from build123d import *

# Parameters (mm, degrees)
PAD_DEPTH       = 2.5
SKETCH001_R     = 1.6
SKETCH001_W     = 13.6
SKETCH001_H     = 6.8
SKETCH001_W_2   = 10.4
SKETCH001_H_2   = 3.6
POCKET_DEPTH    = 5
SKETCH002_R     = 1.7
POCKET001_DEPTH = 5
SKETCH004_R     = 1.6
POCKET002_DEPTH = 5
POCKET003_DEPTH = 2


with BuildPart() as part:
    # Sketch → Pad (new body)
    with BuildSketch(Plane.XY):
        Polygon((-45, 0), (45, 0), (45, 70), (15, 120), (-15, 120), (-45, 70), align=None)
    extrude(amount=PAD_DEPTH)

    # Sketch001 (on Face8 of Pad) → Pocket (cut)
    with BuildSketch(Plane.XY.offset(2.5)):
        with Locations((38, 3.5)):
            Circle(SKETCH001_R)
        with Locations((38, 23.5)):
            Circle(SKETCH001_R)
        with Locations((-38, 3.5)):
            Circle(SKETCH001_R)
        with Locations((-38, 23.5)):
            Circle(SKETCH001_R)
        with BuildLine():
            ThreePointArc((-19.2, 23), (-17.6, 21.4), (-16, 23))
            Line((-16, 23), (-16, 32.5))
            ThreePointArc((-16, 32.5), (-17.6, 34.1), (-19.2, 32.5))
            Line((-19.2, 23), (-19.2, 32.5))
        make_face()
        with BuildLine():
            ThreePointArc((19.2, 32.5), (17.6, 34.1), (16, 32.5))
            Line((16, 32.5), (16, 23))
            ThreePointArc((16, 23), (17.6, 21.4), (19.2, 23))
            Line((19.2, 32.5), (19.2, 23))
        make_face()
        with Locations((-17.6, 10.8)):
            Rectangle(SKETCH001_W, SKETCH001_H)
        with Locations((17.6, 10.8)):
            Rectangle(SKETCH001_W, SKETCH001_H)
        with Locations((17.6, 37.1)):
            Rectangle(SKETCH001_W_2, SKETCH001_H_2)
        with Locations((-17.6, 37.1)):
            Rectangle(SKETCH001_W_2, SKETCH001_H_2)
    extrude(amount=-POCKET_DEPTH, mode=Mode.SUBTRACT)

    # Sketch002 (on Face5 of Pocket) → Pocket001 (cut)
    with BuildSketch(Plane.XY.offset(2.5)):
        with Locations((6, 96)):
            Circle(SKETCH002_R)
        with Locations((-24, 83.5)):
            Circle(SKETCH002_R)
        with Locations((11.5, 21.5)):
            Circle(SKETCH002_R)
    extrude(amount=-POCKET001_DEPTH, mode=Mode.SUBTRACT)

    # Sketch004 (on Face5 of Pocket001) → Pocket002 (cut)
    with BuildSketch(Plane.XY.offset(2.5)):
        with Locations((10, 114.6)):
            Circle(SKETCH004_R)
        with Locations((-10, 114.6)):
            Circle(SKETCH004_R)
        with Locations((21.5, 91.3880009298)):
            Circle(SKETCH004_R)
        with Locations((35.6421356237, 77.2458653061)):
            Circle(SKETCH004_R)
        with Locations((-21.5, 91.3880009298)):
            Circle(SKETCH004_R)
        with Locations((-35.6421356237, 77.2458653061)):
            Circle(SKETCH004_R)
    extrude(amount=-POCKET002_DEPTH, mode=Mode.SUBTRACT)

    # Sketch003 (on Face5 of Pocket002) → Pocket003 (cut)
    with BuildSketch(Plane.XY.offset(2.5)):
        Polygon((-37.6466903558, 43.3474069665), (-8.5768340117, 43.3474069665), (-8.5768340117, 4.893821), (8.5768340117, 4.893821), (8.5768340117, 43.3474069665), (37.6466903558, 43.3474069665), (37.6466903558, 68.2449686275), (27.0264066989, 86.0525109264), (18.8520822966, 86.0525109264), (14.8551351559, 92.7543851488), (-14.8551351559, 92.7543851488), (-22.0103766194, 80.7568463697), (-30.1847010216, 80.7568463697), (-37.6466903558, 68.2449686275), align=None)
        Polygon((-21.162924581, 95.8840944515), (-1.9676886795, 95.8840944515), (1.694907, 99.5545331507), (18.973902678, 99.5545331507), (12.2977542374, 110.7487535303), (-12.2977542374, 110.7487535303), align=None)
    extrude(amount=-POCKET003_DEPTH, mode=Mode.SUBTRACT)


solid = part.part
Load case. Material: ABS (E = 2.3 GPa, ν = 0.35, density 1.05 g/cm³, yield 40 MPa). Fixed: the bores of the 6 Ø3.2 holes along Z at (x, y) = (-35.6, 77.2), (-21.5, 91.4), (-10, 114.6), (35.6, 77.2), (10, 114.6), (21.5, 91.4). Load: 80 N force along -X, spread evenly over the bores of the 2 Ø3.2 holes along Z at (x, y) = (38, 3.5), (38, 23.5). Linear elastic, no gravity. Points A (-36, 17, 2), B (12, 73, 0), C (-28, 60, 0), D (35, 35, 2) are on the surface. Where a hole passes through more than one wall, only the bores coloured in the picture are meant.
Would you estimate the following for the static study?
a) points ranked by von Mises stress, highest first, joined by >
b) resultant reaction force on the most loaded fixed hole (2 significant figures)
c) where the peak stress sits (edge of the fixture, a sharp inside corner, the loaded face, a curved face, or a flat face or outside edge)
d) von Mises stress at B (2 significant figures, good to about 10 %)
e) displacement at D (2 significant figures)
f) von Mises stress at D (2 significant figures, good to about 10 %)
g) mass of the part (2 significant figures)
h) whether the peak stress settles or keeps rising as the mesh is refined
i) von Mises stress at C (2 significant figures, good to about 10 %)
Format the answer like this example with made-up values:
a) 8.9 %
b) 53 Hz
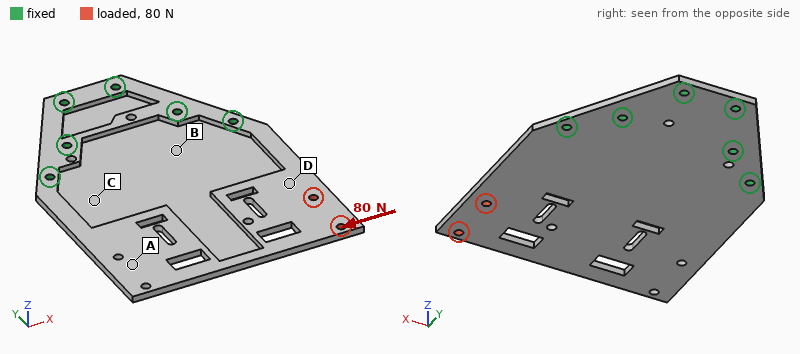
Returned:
a) C > B > D > A
b) 72 N
c) edge of the fixture
d) 3.0 MPa
e) 0.52 mm
f) 1.7 MPa
g) 14 g
h) keeps rising
i) 4.4 MPa
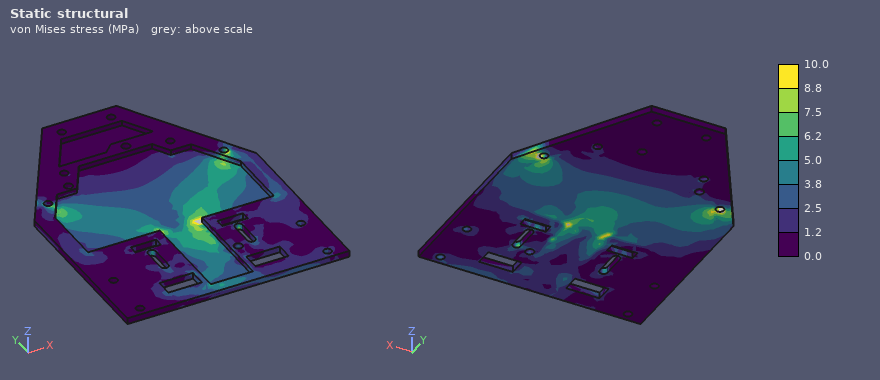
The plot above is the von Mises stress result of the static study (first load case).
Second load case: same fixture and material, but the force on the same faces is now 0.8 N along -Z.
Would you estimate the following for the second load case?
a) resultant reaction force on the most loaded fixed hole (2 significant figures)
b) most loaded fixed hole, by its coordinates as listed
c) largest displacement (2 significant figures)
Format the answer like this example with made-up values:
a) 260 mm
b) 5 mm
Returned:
a) 5.1 N
b) (35.6, 77.2)
c) 1.6 mm
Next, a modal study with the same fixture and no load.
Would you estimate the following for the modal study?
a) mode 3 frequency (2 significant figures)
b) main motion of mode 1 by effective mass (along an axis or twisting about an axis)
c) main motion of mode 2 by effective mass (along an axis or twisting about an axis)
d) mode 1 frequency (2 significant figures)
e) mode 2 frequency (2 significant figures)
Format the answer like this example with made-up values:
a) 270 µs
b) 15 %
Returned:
a) 280 Hz
b) along Z
c) twisting about Y
d) 58 Hz
e) 140 Hz
